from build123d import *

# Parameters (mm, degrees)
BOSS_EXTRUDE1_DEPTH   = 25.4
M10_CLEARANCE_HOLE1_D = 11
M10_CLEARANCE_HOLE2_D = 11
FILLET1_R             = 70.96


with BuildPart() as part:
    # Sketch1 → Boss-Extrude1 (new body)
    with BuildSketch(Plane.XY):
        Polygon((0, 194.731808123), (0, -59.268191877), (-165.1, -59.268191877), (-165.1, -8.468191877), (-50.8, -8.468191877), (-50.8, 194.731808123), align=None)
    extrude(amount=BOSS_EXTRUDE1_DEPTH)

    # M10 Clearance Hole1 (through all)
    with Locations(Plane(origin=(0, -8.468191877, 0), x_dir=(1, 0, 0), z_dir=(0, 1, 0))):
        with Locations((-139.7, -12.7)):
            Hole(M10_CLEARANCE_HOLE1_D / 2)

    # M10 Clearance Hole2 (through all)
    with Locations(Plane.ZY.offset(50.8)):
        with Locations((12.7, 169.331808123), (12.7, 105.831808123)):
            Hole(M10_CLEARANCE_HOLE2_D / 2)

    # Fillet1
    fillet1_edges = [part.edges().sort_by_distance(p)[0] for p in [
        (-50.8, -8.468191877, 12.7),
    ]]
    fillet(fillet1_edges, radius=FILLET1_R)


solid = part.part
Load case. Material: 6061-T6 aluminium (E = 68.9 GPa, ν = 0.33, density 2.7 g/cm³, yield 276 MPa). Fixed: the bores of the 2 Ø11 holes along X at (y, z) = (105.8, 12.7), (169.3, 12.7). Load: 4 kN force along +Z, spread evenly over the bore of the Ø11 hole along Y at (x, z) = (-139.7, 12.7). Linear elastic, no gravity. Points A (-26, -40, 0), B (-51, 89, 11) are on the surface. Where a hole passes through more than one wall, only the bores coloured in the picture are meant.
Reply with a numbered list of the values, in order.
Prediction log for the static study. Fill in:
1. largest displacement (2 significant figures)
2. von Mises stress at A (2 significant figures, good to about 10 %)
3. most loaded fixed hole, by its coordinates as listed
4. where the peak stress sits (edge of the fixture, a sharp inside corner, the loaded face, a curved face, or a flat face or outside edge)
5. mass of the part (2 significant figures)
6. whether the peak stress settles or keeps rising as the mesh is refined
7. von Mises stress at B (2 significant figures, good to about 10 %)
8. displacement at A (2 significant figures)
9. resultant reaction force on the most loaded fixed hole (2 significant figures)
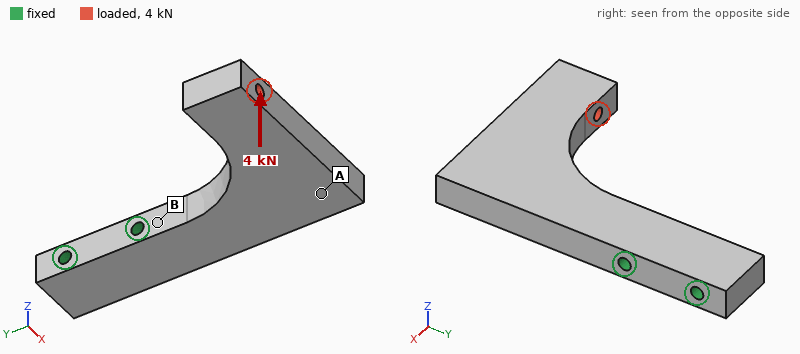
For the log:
1. 2.5 mm
2. 23 MPa
3. (105.8, 12.7)
4. edge of the fixture
5. 1.3 kg
6. keeps rising
7. 82 MPa
8. 0.83 mm
9. 6.4 kN
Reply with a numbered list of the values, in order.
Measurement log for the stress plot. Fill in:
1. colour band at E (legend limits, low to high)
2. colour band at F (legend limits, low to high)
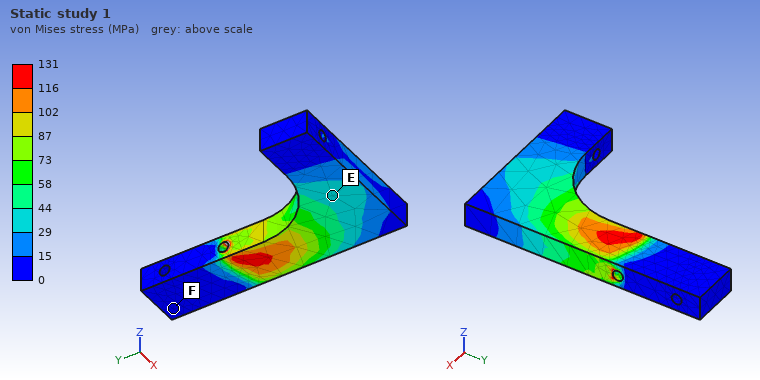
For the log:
1. 29 to 44 MPa
2. 0 to 15 MPa
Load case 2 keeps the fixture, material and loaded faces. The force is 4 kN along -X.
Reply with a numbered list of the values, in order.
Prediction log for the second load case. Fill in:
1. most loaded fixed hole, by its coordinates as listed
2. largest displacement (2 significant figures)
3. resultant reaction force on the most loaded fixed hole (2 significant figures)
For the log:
1. (105.8, 12.7)
2. 0.35 mm
3. 4.4 kN
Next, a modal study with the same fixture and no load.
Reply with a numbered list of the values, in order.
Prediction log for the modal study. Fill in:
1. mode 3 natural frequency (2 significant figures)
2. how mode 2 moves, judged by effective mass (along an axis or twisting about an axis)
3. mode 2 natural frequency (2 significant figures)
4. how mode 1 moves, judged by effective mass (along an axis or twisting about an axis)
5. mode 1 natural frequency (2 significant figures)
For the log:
1. 960 Hz
2. along X
3. 750 Hz
4. along Z
5. 380 Hz
